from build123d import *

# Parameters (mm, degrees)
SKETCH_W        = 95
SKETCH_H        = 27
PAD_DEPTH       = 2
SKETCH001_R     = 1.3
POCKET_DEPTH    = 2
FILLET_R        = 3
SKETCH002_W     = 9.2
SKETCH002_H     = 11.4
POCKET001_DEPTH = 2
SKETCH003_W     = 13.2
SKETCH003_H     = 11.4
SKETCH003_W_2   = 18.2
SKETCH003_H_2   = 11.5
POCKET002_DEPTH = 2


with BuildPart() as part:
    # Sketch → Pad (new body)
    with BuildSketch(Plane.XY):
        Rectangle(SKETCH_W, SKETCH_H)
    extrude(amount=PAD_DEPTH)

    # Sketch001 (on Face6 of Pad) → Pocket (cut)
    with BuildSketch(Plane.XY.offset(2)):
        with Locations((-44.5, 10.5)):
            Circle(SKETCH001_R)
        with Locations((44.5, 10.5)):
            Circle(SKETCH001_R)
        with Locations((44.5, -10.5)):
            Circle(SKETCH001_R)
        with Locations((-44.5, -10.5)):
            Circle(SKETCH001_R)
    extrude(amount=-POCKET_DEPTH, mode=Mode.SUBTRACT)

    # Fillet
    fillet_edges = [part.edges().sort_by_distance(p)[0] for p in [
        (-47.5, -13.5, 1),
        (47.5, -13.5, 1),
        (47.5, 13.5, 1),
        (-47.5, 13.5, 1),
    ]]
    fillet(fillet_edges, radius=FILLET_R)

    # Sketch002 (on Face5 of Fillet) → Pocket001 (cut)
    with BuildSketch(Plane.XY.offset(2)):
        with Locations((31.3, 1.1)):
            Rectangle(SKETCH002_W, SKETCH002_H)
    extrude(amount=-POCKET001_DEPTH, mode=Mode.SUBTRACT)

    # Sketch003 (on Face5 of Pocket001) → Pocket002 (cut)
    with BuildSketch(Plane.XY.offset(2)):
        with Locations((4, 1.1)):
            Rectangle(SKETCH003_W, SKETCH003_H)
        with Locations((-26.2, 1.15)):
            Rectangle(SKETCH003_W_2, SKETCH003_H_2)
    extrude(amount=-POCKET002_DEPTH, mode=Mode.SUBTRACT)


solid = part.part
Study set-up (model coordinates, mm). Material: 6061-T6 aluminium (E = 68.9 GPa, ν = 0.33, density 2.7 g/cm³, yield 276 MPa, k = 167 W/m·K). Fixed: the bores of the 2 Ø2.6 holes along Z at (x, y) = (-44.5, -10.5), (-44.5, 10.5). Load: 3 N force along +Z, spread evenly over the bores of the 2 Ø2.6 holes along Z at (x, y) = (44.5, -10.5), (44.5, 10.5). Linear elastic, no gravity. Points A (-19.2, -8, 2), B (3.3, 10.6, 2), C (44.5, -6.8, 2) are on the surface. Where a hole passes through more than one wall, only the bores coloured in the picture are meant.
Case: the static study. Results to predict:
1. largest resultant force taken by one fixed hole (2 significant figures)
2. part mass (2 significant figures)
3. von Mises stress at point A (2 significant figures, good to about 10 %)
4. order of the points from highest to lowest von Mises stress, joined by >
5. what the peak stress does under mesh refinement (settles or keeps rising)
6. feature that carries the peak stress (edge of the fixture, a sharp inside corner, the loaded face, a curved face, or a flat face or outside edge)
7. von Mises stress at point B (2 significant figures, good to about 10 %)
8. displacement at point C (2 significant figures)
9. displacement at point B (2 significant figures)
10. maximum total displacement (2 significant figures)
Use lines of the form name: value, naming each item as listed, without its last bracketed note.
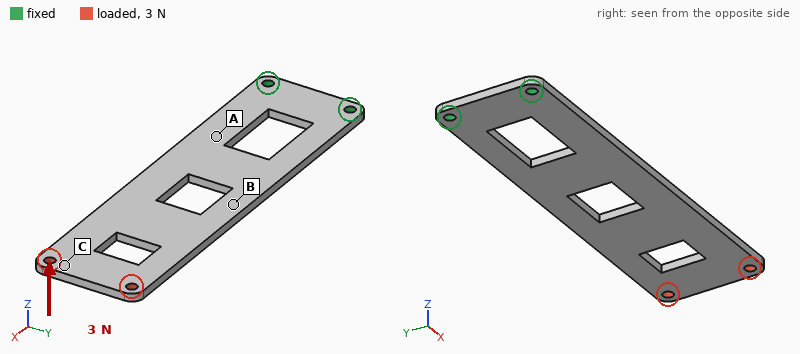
largest resultant force taken by one fixed hole: 1.6 N
part mass: 11 g
von Mises stress at point A: 18 MPa
order of the points from highest to lowest von Mises stress, joined by >: A > B > C
what the peak stress does under mesh refinement: keeps rising
feature that carries the peak stress: edge of the fixture
von Mises stress at point B: 12 MPa
displacement at point C: 0.86 mm
displacement at point B: 0.30 mm
maximum total displacement: 0.90 mm
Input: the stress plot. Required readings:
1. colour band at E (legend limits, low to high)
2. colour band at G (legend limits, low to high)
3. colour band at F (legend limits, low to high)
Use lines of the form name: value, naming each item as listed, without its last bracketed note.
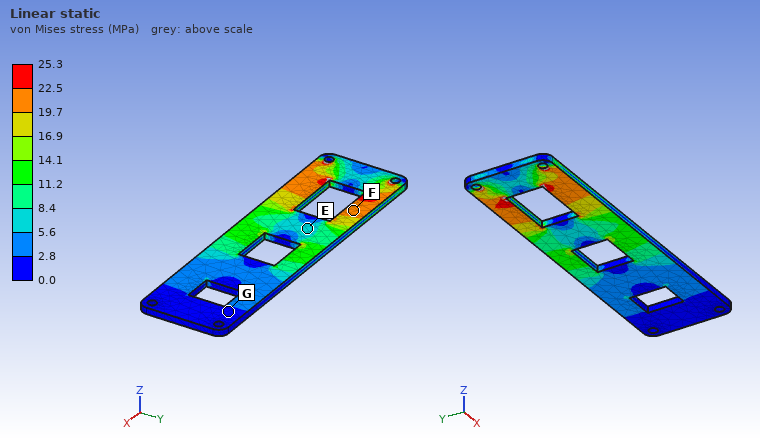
colour band at E: 5.6 to 8.4 MPa
colour band at G: 0.0 to 2.8 MPa
colour band at F: 19.7 to 22.5 MPa
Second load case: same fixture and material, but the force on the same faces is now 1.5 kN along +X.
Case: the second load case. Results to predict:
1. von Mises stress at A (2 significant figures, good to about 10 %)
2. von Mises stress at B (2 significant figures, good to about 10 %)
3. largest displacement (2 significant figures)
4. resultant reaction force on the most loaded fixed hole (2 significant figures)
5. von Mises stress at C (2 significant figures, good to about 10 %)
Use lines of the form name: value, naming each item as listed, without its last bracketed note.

von Mises stress at A: 44 MPa
von Mises stress at B: 51 MPa
largest displacement: 72 µm
resultant reaction force on the most loaded fixed hole: 760 N
von Mises stress at C: 22 MPa
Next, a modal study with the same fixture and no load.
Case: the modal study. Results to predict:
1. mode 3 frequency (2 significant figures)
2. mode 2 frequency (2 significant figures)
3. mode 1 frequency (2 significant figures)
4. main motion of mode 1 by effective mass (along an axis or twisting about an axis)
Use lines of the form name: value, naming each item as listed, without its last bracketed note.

mode 3 frequency: 1100 Hz
mode 2 frequency: 1100 Hz
mode 1 frequency: 170 Hz
main motion of mode 1 by effective mass: along Z
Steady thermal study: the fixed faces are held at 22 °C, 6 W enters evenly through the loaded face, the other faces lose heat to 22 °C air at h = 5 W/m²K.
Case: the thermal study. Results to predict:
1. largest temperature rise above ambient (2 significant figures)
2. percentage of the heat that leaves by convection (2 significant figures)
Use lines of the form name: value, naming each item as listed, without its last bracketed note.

largest temperature rise above ambient: 82 K
percentage of the heat that leaves by convection: 16 %
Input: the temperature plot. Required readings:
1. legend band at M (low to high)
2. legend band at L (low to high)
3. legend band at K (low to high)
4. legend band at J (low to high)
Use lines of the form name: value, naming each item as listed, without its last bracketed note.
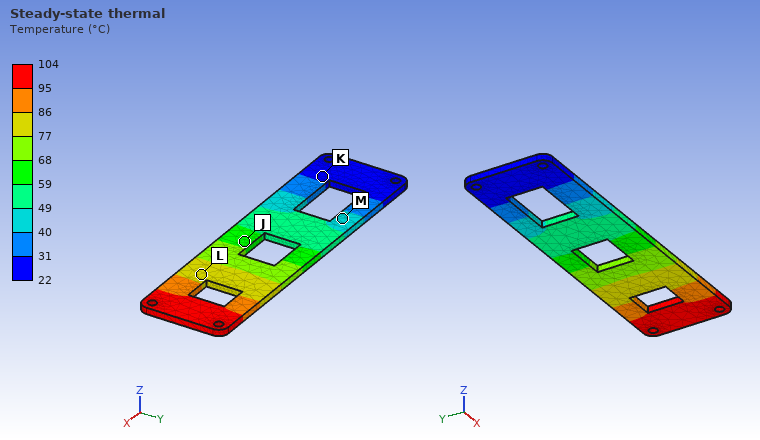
legend band at M: 40 to 49 °C
legend band at L: 77 to 86 °C
legend band at K: 22 to 31 °C
legend band at J: 59 to 68 °C
